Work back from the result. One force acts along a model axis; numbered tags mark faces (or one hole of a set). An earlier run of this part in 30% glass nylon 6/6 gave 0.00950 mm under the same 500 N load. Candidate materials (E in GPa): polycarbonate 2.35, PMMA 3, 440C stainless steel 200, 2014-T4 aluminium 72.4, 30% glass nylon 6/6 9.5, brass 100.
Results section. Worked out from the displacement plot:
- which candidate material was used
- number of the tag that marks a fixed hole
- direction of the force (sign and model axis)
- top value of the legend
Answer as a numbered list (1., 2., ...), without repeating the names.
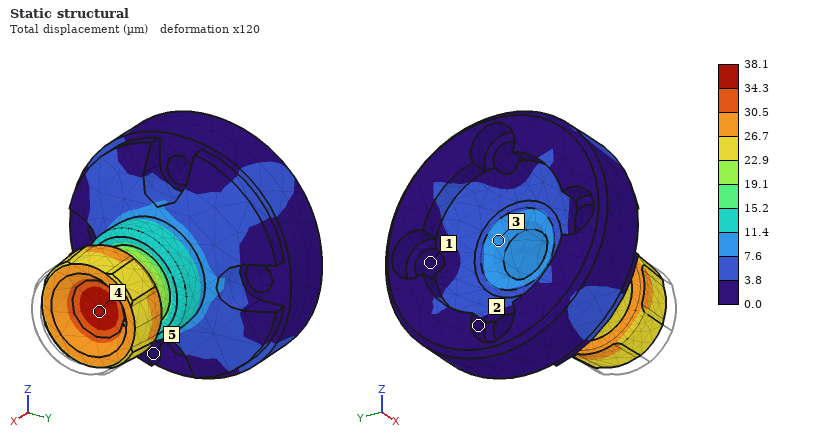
1. polycarbonate
2. 1
3. -X
4. 38.1 µm
